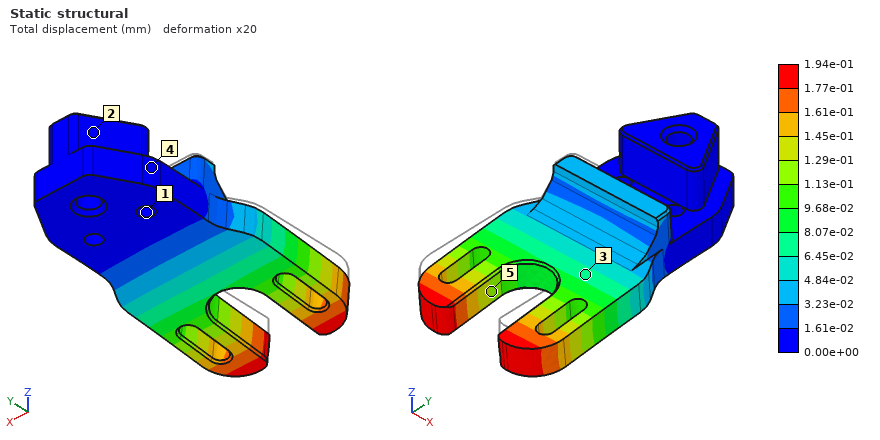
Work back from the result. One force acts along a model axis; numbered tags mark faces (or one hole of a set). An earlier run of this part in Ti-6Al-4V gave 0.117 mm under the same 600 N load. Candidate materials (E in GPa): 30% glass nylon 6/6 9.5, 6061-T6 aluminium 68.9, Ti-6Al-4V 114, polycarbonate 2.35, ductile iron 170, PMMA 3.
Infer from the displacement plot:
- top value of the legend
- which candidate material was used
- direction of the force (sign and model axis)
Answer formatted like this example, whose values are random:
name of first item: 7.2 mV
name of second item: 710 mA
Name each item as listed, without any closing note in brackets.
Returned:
top value of the legend: 1.94e-01 mm
which candidate material was used: 6061-T6 aluminium
direction of the force: -Z
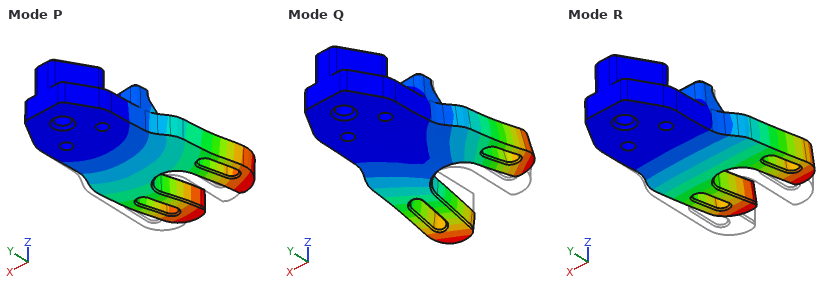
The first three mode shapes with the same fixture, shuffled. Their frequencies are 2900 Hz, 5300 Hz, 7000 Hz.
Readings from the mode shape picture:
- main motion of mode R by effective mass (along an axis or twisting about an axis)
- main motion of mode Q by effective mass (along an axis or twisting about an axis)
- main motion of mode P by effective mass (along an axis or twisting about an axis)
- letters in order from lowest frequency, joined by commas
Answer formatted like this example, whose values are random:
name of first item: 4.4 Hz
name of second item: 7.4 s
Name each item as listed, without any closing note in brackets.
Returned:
main motion of mode R by effective mass: along Z
main motion of mode Q by effective mass: twisting about Y
main motion of mode P by effective mass: along X
letters in order from lowest frequency, joined by commas: R, Q, P
